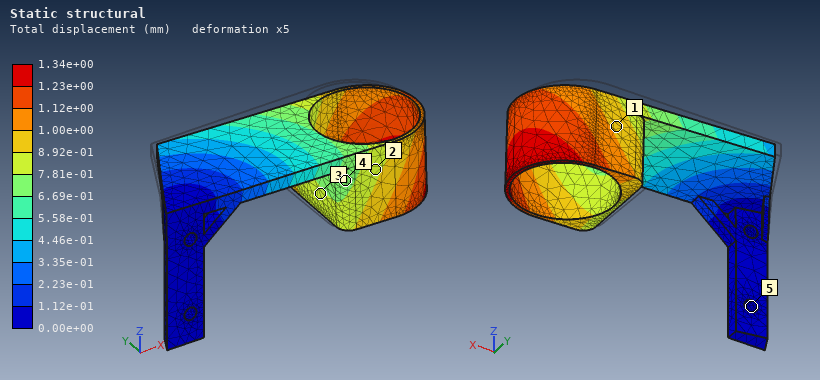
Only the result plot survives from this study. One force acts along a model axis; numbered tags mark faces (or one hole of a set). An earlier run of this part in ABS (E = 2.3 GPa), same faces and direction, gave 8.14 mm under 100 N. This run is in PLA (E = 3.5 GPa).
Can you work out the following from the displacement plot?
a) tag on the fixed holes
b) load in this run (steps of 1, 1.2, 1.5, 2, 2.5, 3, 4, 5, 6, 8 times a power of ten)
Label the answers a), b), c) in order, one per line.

a) 5
b) 25 N
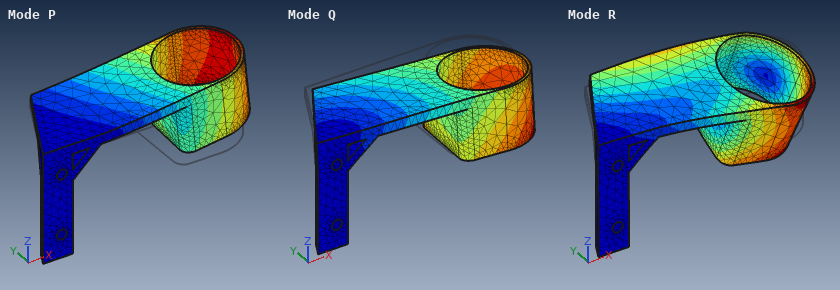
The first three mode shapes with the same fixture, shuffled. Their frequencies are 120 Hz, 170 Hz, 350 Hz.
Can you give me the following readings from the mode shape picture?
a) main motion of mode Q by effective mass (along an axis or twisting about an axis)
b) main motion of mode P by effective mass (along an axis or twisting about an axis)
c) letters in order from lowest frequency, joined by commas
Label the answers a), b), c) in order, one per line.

a) along Y
b) along Z
c) P, Q, R
